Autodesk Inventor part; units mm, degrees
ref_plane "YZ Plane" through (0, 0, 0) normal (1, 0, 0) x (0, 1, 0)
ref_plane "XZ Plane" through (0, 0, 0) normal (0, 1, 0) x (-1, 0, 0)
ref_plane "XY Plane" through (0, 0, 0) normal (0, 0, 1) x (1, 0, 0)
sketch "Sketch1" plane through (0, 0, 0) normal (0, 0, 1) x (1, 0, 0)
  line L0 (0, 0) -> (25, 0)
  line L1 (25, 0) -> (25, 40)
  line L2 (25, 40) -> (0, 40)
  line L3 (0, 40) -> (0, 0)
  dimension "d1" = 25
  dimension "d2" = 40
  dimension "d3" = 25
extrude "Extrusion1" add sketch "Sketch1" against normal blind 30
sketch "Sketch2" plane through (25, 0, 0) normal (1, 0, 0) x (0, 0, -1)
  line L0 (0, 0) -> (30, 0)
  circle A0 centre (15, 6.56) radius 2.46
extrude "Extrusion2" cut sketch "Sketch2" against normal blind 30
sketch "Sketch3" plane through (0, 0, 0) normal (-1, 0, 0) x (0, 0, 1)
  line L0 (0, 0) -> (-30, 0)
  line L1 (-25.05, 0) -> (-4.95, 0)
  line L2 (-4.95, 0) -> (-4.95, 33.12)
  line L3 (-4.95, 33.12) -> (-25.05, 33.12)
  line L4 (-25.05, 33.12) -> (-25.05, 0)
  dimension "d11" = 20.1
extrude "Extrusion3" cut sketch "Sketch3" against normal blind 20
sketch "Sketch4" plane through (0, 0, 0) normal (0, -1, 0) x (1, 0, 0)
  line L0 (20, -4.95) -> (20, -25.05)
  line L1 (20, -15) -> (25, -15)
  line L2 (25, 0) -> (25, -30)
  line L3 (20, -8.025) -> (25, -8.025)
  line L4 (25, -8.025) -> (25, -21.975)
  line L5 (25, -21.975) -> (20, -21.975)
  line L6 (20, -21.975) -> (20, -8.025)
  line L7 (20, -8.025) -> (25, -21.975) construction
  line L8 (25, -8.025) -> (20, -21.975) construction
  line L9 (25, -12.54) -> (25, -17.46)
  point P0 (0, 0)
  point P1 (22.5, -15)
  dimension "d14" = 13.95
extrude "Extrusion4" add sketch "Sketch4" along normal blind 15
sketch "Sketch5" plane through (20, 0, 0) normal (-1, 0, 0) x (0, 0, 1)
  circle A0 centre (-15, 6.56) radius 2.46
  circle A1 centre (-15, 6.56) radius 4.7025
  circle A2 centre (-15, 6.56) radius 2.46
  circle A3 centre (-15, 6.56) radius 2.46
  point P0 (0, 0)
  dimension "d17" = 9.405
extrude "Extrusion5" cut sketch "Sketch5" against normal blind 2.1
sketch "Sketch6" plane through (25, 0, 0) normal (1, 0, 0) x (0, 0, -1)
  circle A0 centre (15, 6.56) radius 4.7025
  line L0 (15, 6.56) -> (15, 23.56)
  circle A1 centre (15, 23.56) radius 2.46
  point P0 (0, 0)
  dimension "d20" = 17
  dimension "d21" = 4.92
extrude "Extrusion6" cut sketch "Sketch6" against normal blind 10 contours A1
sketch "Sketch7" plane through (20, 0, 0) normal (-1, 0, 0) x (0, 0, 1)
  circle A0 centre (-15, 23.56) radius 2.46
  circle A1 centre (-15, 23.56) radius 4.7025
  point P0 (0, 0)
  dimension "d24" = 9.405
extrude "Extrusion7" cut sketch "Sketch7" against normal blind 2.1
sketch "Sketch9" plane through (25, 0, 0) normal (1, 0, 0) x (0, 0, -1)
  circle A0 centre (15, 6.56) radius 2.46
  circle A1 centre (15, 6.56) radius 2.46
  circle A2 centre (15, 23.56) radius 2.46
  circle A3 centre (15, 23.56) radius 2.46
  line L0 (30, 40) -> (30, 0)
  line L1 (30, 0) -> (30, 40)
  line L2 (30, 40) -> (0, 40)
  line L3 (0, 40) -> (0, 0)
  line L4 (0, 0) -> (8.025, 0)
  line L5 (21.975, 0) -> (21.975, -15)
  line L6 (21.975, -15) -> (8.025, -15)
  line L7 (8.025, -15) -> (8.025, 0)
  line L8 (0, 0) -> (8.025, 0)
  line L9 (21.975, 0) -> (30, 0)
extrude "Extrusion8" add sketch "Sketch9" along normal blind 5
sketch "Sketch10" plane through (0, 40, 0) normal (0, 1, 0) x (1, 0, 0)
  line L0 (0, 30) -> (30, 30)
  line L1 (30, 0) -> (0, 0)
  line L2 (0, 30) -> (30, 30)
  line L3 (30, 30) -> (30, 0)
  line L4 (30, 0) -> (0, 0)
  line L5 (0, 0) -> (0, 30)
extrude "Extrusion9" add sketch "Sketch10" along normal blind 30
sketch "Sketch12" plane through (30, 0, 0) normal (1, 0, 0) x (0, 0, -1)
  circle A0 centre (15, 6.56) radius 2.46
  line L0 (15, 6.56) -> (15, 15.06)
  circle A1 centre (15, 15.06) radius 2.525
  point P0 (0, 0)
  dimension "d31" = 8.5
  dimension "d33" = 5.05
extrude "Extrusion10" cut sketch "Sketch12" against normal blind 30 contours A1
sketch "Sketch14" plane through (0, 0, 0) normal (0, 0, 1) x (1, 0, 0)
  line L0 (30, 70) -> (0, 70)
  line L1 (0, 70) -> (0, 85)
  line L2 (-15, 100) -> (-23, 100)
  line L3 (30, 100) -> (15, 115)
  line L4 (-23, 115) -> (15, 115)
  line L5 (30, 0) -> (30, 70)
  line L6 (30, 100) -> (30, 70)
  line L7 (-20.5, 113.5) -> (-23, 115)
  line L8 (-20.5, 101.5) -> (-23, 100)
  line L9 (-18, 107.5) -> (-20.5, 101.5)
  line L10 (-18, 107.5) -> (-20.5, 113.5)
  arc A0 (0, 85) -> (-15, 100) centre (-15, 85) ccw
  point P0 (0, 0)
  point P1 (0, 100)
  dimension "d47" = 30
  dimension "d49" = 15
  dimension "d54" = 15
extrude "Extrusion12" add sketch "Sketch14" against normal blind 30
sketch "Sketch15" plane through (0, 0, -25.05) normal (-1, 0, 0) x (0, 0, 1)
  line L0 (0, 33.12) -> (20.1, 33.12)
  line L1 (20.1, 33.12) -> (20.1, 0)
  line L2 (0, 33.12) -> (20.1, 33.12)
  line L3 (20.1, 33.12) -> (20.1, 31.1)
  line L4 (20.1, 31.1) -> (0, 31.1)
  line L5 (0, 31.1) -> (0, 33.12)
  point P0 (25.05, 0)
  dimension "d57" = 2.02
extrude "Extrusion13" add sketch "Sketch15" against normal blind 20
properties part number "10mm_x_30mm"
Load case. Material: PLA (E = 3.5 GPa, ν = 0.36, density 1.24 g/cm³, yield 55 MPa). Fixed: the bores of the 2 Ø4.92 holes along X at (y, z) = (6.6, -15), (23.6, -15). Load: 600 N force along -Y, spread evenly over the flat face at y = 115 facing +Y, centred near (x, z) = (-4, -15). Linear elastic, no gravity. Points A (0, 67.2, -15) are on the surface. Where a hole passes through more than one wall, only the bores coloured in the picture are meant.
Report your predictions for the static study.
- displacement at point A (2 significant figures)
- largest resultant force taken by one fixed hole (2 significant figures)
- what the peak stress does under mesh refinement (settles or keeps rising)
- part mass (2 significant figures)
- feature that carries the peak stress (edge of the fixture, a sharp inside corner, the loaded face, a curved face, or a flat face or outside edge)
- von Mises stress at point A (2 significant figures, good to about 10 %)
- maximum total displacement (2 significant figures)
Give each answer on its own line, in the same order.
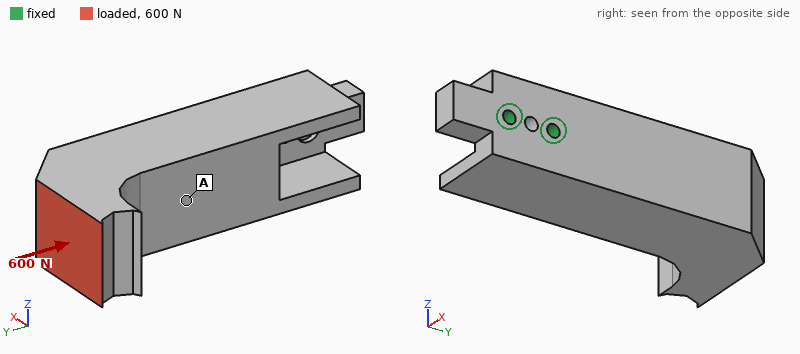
0.44 mm
800 N
keeps rising
120 g
edge of the fixture
3.2 MPa
1.0 mm
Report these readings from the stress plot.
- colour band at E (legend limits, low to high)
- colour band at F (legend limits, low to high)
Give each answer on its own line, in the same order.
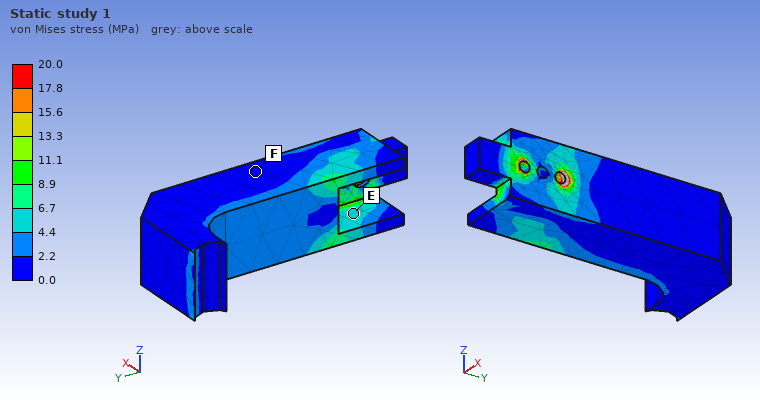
4.4 to 6.7 MPa
0.0 to 2.2 MPa
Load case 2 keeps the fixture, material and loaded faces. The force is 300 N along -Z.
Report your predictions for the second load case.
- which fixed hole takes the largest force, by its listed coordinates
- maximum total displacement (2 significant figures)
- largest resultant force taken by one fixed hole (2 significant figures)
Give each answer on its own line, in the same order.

(23.6, -15)
1.4 mm
1.5 kN
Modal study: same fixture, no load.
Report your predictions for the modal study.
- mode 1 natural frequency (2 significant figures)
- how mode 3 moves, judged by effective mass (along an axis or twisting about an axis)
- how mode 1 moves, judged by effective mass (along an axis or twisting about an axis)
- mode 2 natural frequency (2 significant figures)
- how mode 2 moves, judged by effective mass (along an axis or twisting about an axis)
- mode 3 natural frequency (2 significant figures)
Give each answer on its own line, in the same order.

360 Hz
twisting about Y
along X
420 Hz
along Z
1000 Hz
